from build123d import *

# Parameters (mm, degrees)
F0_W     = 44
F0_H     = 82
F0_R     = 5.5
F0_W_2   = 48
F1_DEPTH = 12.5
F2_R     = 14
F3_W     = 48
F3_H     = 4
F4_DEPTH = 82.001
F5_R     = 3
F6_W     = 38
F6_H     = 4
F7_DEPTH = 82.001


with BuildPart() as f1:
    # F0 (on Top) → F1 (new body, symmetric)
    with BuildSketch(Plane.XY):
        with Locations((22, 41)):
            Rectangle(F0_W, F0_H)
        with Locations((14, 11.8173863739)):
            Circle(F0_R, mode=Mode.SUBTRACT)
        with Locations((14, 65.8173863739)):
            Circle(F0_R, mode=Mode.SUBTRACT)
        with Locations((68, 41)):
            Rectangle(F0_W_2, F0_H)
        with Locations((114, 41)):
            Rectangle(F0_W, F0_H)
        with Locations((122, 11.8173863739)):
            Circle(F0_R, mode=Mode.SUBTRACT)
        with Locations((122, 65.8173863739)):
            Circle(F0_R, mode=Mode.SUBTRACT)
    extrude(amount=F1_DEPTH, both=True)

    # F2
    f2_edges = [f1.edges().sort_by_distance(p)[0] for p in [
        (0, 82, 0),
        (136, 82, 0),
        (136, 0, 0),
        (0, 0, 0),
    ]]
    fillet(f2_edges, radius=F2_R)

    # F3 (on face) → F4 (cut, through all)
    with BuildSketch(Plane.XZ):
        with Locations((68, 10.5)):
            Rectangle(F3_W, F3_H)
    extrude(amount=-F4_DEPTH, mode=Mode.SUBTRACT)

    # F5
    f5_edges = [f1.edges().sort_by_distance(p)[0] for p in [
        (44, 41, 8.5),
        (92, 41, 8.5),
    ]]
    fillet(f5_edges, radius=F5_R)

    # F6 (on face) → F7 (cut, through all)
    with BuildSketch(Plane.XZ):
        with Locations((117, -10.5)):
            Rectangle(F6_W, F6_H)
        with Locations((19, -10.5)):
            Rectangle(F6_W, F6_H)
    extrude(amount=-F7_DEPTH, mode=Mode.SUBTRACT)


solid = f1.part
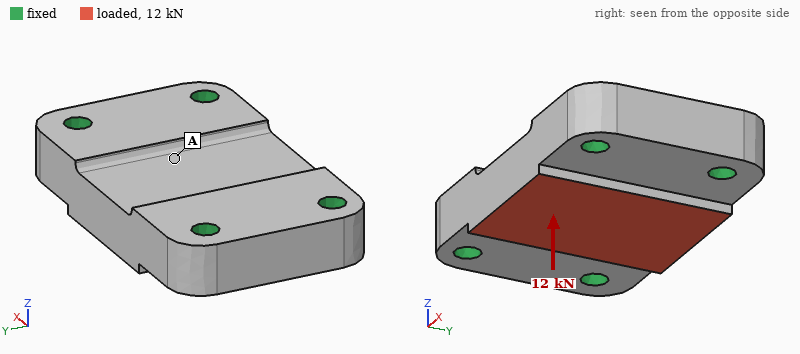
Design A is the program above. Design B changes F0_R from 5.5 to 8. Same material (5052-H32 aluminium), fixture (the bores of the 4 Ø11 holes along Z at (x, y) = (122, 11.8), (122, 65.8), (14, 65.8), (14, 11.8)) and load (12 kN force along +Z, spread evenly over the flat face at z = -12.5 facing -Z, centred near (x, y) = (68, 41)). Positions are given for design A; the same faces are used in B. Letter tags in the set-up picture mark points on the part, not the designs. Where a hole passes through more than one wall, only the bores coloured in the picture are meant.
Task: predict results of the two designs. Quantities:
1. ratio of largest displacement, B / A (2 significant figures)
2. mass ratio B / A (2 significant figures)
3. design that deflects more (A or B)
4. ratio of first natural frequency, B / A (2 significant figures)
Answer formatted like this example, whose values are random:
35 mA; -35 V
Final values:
0.81; 0.96; A; 1.1
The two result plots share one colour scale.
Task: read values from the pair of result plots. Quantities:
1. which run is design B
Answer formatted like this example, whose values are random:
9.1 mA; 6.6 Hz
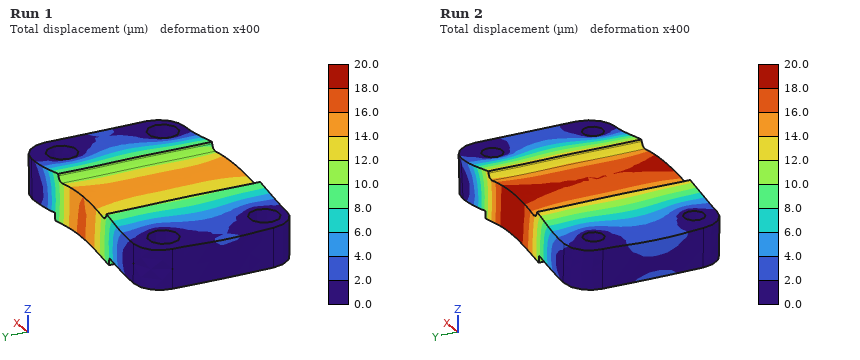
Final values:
Run 1
